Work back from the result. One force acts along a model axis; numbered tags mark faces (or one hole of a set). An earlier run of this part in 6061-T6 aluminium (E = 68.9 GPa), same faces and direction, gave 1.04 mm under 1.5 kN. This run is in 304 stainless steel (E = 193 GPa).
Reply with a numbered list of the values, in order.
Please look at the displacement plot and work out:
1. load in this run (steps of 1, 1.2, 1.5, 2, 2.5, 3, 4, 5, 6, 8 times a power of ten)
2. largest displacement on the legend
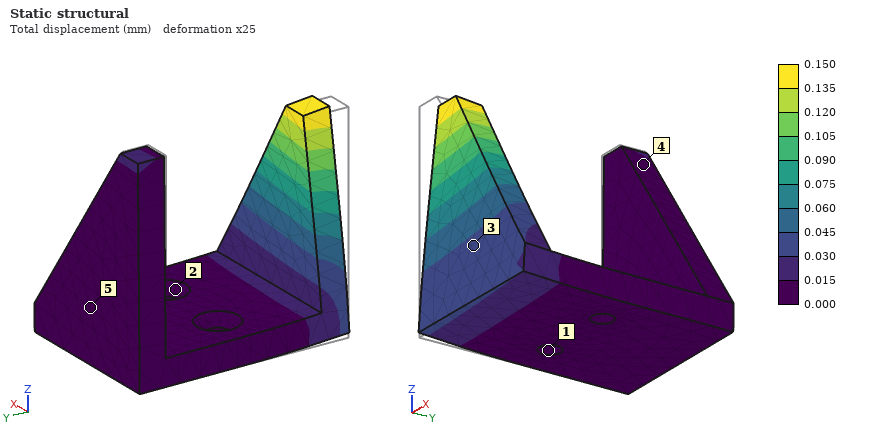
1. 600 N
2. 0.150 mm
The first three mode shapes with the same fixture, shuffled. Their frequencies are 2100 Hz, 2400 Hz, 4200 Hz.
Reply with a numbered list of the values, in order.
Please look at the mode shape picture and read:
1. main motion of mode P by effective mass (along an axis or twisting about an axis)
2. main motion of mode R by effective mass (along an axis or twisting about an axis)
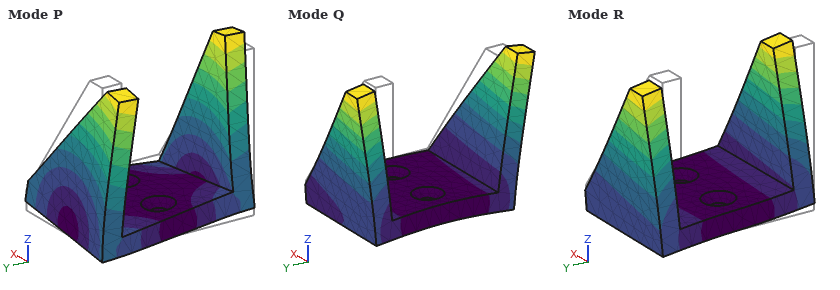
1. twisting about Z
2. along Y
